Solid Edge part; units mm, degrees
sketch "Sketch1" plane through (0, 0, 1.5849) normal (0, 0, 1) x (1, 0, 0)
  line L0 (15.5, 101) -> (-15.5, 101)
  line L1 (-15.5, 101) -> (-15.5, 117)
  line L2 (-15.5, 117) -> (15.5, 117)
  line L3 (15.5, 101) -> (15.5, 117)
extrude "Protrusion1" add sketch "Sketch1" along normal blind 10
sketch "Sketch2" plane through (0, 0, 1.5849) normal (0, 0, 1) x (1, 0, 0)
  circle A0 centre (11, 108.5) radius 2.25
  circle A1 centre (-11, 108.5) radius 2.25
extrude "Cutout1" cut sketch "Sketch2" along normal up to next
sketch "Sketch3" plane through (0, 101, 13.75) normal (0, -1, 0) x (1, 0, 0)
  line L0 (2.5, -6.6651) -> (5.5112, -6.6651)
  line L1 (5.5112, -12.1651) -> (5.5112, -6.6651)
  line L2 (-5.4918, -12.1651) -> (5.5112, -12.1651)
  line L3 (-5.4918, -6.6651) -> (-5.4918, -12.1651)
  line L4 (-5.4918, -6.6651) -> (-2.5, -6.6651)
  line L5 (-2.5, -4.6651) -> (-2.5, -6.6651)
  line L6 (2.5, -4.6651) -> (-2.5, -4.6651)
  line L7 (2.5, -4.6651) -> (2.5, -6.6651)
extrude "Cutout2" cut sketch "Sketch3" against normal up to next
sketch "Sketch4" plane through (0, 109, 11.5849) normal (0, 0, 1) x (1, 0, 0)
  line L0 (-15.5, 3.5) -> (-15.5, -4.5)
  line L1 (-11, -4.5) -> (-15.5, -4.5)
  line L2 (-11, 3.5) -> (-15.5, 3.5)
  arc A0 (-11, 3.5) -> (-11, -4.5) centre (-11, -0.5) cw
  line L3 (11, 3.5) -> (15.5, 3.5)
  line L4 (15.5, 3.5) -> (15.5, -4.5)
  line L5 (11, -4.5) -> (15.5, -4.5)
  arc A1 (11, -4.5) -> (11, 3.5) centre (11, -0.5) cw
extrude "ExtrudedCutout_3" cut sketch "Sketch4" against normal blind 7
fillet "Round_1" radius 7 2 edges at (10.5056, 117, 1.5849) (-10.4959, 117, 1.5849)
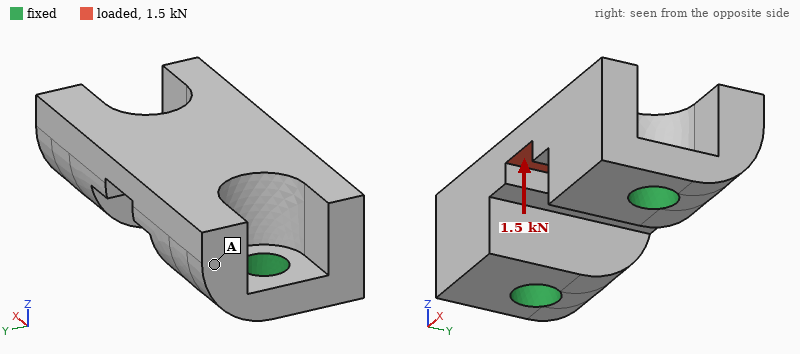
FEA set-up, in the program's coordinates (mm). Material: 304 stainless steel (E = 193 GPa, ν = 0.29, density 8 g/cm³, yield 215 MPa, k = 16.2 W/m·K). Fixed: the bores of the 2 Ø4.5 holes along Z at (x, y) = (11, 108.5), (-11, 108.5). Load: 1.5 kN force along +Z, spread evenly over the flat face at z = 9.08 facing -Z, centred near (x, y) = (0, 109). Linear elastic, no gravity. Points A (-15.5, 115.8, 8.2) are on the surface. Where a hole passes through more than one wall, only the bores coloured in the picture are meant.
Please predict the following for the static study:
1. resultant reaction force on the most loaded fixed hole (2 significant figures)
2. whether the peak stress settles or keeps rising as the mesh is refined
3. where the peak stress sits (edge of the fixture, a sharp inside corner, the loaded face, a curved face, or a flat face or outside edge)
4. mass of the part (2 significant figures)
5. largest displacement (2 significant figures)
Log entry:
1.0 kN
keeps rising
edge of the fixture
21 g
5.7 µm
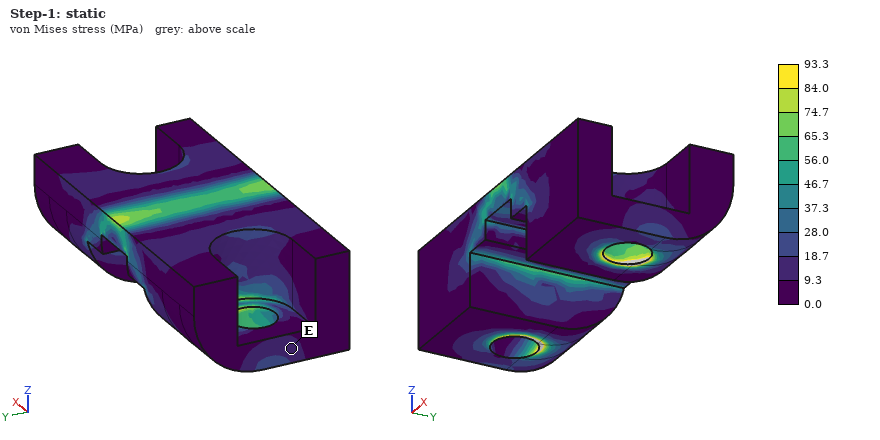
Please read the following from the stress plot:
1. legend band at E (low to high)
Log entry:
9.3 to 18.7 MPa
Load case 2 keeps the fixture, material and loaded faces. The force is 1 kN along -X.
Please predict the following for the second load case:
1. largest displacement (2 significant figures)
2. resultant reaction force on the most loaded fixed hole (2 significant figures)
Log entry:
3.3 µm
530 N
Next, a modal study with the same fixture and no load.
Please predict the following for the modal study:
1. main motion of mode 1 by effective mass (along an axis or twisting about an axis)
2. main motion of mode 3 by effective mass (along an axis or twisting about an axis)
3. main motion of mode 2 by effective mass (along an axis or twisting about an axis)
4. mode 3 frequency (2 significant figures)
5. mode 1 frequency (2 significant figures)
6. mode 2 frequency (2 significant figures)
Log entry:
along Y
along X
twisting about Z
28 kHz
16 kHz
24 kHz
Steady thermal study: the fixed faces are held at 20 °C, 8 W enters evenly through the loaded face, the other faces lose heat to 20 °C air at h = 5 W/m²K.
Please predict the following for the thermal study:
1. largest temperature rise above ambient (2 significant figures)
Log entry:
60 K
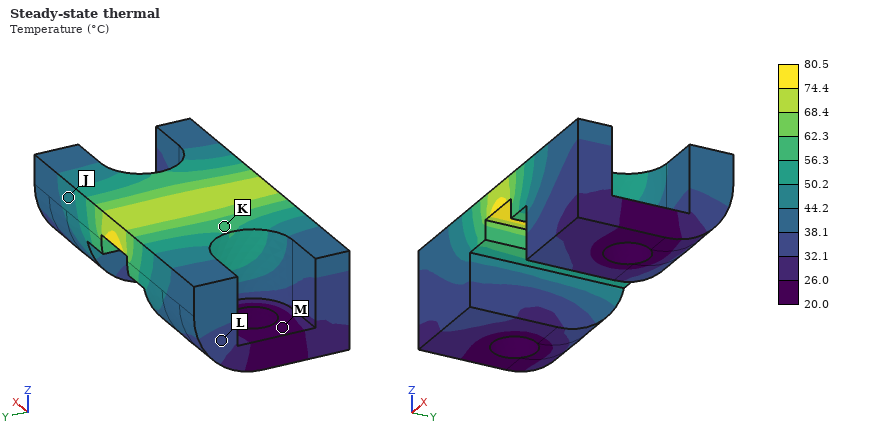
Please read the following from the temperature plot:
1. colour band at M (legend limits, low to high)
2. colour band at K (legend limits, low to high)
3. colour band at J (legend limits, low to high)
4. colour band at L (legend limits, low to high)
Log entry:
20.0 to 26.0 °C
56.3 to 62.3 °C
44.2 to 50.2 °C
32.1 to 38.1 °C
